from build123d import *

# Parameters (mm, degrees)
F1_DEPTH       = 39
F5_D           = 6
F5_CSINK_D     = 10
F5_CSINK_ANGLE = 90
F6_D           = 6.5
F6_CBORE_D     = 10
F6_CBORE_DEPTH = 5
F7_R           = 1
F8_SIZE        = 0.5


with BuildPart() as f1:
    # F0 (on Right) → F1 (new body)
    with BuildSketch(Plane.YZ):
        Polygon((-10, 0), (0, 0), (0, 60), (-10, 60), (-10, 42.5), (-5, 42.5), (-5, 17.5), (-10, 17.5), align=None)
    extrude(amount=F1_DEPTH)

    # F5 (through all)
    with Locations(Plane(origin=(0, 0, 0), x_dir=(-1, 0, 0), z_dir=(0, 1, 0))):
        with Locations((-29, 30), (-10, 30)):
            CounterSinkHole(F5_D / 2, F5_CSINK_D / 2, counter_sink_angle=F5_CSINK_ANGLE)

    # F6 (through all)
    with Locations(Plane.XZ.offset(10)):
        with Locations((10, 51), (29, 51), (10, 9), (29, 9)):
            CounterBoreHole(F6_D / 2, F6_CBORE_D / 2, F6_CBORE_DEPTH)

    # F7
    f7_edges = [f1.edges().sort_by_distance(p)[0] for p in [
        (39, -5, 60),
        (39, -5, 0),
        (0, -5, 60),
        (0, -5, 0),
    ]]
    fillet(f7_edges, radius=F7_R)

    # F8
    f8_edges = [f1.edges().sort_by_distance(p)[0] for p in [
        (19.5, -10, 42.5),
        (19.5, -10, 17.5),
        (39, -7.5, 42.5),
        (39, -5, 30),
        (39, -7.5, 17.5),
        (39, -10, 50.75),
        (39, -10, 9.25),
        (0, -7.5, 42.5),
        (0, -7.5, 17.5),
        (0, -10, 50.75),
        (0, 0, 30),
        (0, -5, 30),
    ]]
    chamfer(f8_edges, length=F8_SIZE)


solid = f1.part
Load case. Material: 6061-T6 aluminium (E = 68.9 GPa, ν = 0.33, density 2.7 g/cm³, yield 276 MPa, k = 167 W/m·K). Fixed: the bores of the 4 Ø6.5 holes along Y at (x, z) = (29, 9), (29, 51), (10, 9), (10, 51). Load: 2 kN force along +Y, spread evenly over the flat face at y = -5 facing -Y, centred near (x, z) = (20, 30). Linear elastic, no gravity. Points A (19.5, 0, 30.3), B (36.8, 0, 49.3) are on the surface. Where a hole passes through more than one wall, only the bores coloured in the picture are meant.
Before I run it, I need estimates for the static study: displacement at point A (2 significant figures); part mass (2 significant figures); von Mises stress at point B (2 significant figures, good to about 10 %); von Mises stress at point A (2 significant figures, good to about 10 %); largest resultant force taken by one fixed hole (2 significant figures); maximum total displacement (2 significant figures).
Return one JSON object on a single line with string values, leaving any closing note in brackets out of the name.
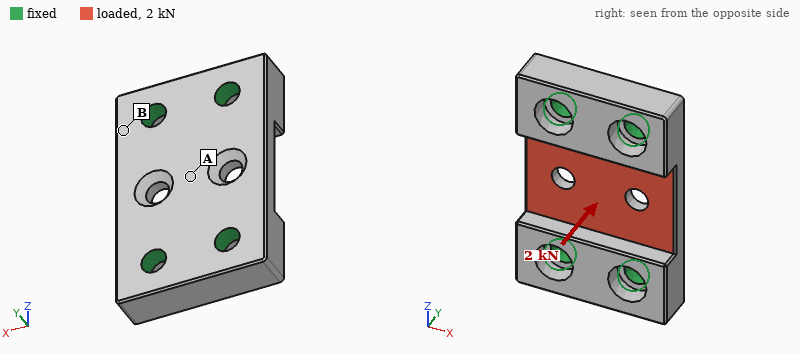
{"displacement at point A": "15 µm", "part mass": "43 g", "von Mises stress at point B": "11 MPa", "von Mises stress at point A": "27 MPa", "largest resultant force taken by one fixed hole": "500 N", "maximum total displacement": "16 µm"}
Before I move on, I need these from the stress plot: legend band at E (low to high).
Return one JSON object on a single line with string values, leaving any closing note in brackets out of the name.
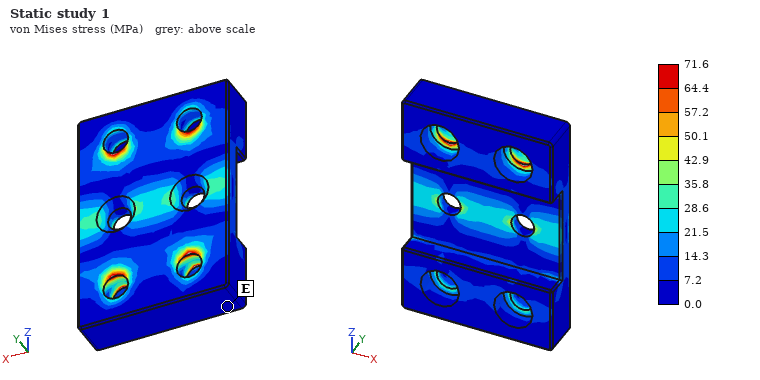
{"legend band at E": "0.0 to 7.2 MPa"}
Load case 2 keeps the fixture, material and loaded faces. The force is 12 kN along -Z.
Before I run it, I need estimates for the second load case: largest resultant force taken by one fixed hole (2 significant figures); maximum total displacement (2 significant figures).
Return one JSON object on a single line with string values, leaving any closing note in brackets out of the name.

{"largest resultant force taken by one fixed hole": "3.1 kN", "maximum total displacement": "8.3 µm"}
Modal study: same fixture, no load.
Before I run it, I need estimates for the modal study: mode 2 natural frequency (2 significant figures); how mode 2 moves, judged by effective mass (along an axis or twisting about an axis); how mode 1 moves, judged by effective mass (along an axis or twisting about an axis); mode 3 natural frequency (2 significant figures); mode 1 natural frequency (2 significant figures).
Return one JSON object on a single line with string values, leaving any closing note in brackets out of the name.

{"mode 2 natural frequency": "20 kHz", "how mode 2 moves, judged by effective mass": "twisting about Z", "how mode 1 moves, judged by effective mass": "along Y", "mode 3 natural frequency": "30 kHz", "mode 1 natural frequency": "17 kHz"}
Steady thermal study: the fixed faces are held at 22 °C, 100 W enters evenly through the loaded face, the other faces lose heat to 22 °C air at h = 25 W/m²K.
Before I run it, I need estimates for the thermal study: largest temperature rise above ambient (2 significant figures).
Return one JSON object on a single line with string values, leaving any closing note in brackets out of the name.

{"largest temperature rise above ambient": "20 K"}
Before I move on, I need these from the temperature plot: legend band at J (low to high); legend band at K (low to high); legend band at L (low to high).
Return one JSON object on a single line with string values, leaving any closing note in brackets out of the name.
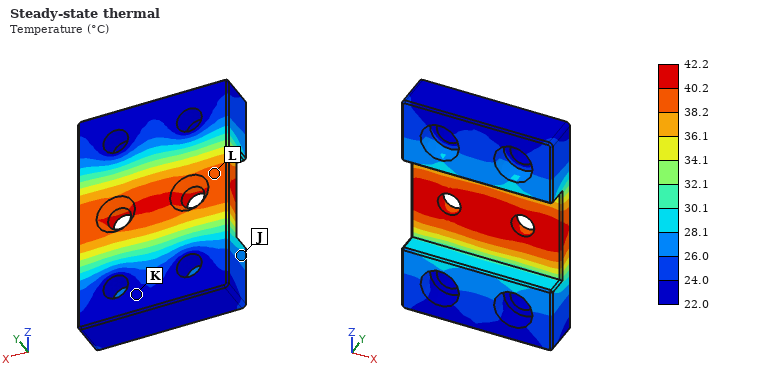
{"legend band at J": "26.0 to 28.1 °C", "legend band at K": "22.0 to 24.0 °C", "legend band at L": "38.2 to 40.2 °C"}
